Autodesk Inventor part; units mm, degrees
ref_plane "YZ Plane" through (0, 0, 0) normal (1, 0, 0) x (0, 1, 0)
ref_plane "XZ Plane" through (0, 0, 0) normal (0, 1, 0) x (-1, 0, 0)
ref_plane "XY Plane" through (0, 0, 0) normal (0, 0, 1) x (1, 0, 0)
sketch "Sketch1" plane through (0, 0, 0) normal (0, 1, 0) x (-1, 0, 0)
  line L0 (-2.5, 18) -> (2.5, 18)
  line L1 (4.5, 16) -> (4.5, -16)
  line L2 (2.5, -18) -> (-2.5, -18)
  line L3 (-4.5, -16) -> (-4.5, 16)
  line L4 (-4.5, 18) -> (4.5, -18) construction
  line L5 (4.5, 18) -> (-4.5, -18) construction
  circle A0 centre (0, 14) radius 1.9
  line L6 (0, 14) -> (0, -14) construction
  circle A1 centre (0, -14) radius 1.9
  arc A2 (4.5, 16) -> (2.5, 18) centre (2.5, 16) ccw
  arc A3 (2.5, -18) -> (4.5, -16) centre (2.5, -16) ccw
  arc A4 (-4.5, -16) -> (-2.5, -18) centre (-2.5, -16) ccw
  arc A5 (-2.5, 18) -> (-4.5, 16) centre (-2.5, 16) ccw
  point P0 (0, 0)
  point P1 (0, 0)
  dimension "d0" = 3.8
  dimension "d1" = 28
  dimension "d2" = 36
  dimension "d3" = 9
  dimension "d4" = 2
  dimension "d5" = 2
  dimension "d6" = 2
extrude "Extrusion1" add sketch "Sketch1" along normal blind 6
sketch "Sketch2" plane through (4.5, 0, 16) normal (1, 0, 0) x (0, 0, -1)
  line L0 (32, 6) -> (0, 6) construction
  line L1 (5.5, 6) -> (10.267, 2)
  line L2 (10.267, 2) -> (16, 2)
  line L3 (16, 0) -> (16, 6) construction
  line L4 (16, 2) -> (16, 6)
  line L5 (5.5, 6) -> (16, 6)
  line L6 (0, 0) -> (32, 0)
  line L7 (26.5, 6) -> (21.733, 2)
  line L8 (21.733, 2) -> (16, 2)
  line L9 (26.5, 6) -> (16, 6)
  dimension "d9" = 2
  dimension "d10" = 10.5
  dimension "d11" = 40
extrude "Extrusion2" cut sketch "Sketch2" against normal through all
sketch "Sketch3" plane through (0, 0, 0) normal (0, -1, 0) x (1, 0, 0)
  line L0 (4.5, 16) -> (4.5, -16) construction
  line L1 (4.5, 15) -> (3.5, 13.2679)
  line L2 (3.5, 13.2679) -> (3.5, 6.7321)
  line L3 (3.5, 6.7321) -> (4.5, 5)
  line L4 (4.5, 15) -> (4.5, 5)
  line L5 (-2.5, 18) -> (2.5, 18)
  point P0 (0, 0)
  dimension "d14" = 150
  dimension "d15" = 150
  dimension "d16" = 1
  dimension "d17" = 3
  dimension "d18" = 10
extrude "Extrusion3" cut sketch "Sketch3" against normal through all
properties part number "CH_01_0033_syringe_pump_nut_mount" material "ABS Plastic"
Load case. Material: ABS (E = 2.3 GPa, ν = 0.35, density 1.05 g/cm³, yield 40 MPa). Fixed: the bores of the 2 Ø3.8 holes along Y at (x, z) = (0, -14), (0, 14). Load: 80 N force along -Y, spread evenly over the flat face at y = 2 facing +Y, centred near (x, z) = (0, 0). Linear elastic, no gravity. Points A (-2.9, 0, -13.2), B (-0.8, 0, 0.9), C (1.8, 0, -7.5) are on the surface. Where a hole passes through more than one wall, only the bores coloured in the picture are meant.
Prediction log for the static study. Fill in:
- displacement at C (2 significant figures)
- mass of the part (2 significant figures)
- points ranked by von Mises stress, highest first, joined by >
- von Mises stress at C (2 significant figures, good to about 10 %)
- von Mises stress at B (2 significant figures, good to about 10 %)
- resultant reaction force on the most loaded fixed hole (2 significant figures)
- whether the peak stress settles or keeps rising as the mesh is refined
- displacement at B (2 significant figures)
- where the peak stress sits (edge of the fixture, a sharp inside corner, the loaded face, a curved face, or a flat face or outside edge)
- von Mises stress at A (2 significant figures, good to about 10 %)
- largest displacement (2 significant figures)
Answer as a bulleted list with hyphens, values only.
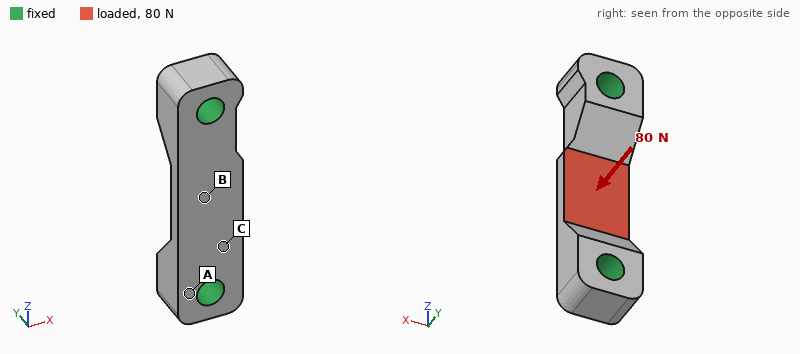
- 0.021 mm
- 1.2 g
- B > C > A
- 5.5 MPa
- 11 MPa
- 53 N
- keeps rising
- 0.089 mm
- a sharp inside corner
- 2.2 MPa
- 0.10 mm
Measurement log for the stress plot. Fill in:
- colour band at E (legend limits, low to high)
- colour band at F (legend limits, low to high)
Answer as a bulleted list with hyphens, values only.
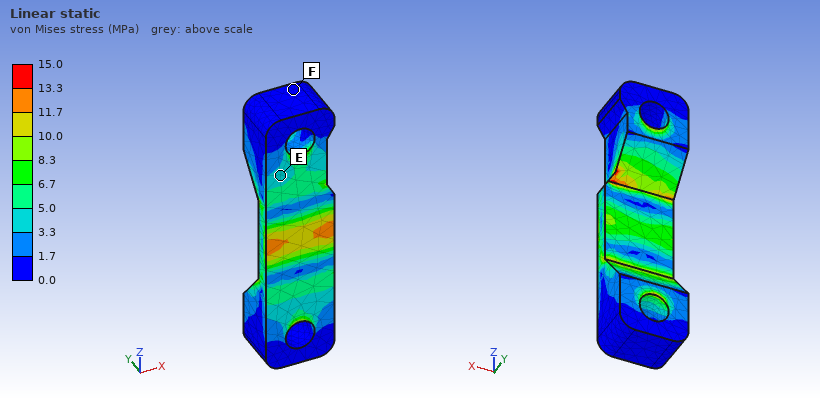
- 3.3 to 5.0 MPa
- 0.0 to 1.7 MPa
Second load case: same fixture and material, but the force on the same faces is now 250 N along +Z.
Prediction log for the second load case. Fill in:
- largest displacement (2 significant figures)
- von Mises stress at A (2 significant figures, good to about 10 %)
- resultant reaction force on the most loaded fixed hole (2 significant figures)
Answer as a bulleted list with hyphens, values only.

- 45 µm
- 4.2 MPa
- 130 N
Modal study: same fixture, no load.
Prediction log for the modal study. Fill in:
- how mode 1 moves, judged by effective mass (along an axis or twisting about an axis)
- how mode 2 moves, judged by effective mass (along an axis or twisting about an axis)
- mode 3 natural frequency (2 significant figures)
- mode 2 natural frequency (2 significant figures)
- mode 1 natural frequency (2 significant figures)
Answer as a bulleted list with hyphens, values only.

- along Y
- along X
- 15 kHz
- 13 kHz
- 11 kHz
